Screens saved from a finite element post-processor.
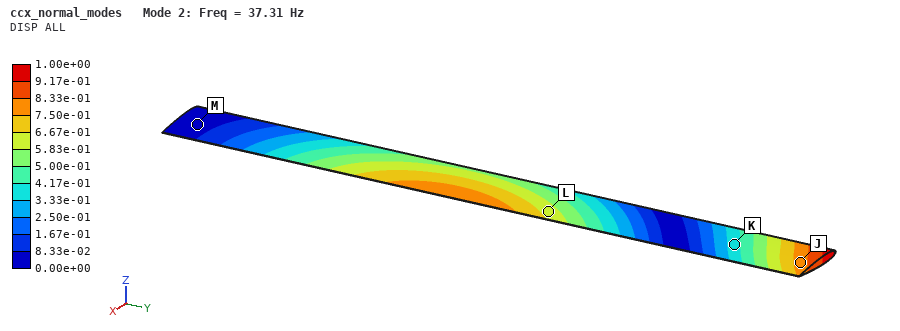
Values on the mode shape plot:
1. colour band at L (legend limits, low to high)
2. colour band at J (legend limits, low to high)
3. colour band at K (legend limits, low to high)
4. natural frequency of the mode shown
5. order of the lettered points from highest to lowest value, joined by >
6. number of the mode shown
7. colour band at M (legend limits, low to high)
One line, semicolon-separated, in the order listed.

5.83e-01 to 6.67e-01; 7.50e-01 to 8.33e-01; 3.33e-01 to 4.17e-01; 37.31 Hz; J > L > K > M; 2; 0.00e+00 to 8.33e-02
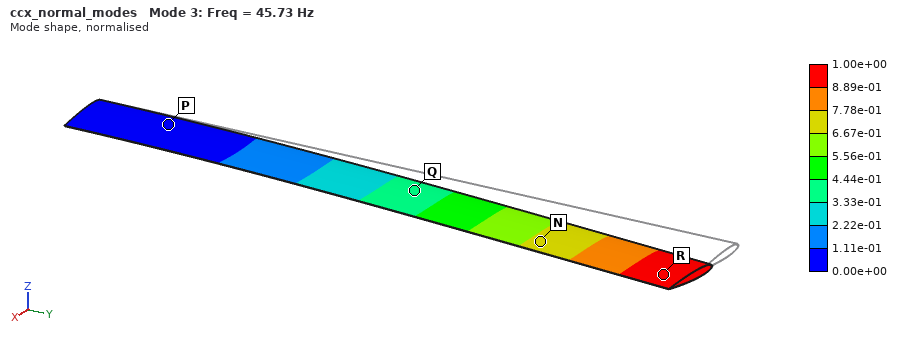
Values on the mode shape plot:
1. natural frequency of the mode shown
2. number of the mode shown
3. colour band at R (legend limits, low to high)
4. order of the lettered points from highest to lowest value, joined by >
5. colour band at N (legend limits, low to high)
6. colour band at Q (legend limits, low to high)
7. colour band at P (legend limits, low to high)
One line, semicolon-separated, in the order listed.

45.73 Hz; 3; 8.89e-01 to 1.00e+00; R > N > Q > P; 6.67e-01 to 7.78e-01; 3.33e-01 to 4.44e-01; 0.00e+00 to 1.11e-01
